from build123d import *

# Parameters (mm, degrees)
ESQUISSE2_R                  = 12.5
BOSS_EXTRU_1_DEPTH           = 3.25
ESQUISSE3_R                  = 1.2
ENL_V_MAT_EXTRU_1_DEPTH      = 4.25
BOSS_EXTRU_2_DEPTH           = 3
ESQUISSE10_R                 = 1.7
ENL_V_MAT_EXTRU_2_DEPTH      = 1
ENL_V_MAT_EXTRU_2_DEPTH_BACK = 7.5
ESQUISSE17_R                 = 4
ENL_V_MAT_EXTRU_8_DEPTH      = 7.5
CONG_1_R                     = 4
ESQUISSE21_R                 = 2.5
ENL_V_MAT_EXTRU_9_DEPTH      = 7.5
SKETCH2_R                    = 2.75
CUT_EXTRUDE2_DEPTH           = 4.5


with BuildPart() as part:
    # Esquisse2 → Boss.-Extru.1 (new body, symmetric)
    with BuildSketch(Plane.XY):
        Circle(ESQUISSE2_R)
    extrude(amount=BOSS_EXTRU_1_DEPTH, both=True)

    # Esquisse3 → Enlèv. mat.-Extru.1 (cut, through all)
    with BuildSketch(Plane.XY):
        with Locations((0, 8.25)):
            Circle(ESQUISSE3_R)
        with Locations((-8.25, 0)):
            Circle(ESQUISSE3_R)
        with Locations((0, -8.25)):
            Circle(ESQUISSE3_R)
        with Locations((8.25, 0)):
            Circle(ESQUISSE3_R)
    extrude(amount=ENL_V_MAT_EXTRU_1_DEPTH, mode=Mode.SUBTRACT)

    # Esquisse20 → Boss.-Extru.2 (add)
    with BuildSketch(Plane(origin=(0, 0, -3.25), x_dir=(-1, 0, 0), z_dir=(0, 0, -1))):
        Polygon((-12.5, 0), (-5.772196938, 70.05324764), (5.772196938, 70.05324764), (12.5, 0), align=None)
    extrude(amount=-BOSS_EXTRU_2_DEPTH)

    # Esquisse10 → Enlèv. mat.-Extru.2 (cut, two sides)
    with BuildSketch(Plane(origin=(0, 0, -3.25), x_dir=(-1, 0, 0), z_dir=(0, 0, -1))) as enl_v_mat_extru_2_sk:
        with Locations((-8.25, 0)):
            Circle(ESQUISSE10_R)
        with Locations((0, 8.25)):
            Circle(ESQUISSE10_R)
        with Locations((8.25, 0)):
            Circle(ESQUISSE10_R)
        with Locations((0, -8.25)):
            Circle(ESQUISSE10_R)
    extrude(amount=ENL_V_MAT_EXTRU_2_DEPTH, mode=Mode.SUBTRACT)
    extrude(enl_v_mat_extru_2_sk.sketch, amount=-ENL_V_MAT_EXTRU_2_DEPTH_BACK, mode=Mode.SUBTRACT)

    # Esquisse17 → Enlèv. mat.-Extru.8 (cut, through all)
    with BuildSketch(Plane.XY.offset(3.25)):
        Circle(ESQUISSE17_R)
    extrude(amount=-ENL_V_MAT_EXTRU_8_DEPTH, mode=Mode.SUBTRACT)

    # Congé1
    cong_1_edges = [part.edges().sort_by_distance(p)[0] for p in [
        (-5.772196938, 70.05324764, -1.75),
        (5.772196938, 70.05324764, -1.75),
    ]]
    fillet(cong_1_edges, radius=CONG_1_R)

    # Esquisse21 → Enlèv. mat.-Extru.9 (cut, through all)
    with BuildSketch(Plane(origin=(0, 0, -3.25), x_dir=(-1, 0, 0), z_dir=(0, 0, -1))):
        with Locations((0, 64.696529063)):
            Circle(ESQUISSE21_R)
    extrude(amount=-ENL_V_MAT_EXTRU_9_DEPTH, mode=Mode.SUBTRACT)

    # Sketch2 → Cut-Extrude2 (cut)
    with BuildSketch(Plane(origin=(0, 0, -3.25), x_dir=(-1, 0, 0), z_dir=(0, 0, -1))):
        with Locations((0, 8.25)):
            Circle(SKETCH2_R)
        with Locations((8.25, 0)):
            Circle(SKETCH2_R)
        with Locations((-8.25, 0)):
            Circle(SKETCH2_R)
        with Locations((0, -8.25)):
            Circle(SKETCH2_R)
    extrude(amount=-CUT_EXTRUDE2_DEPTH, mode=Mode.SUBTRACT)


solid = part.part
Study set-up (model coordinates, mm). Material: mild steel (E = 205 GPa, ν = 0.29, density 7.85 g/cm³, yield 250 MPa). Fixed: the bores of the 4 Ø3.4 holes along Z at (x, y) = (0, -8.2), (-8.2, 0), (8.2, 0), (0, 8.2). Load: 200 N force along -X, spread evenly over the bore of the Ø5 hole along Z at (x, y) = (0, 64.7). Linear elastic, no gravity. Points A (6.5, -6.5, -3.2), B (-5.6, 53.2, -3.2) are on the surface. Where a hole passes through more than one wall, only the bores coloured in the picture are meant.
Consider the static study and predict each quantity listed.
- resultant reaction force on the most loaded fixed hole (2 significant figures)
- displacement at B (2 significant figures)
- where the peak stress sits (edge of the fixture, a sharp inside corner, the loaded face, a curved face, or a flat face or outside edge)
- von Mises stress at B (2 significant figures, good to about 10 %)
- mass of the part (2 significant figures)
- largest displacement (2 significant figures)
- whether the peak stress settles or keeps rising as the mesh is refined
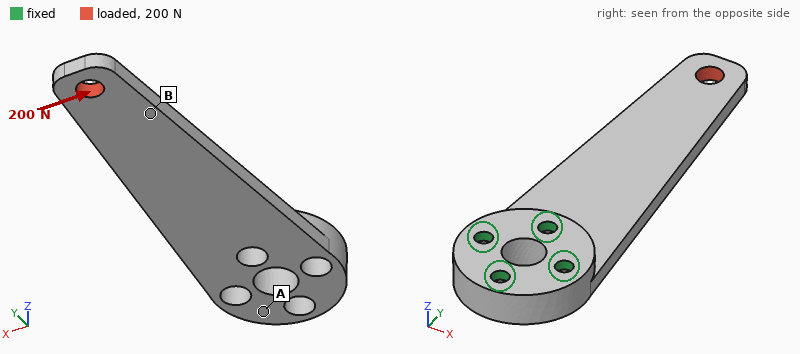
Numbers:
470 N
28 µm
edge of the fixture
17 MPa
42 g
47 µm
keeps rising
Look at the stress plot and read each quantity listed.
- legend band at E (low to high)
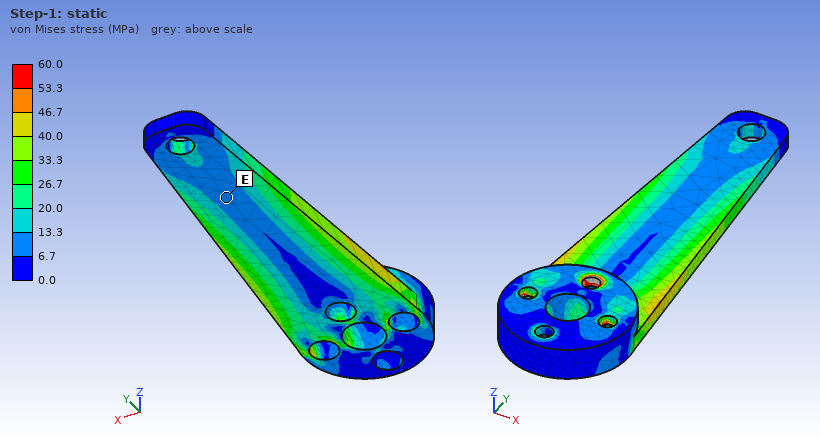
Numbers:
6.7 to 13.3 MPa
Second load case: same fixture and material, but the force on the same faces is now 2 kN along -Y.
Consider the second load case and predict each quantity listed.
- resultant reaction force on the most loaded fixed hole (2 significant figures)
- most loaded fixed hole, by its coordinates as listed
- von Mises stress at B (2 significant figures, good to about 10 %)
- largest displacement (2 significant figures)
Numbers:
770 N
(0, 8.2)
46 MPa
32 µm
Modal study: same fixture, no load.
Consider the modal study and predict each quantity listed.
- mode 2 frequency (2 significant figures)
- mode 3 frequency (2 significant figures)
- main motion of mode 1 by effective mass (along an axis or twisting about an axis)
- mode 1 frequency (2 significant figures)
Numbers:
4500 Hz
4600 Hz
along Z
870 Hz
